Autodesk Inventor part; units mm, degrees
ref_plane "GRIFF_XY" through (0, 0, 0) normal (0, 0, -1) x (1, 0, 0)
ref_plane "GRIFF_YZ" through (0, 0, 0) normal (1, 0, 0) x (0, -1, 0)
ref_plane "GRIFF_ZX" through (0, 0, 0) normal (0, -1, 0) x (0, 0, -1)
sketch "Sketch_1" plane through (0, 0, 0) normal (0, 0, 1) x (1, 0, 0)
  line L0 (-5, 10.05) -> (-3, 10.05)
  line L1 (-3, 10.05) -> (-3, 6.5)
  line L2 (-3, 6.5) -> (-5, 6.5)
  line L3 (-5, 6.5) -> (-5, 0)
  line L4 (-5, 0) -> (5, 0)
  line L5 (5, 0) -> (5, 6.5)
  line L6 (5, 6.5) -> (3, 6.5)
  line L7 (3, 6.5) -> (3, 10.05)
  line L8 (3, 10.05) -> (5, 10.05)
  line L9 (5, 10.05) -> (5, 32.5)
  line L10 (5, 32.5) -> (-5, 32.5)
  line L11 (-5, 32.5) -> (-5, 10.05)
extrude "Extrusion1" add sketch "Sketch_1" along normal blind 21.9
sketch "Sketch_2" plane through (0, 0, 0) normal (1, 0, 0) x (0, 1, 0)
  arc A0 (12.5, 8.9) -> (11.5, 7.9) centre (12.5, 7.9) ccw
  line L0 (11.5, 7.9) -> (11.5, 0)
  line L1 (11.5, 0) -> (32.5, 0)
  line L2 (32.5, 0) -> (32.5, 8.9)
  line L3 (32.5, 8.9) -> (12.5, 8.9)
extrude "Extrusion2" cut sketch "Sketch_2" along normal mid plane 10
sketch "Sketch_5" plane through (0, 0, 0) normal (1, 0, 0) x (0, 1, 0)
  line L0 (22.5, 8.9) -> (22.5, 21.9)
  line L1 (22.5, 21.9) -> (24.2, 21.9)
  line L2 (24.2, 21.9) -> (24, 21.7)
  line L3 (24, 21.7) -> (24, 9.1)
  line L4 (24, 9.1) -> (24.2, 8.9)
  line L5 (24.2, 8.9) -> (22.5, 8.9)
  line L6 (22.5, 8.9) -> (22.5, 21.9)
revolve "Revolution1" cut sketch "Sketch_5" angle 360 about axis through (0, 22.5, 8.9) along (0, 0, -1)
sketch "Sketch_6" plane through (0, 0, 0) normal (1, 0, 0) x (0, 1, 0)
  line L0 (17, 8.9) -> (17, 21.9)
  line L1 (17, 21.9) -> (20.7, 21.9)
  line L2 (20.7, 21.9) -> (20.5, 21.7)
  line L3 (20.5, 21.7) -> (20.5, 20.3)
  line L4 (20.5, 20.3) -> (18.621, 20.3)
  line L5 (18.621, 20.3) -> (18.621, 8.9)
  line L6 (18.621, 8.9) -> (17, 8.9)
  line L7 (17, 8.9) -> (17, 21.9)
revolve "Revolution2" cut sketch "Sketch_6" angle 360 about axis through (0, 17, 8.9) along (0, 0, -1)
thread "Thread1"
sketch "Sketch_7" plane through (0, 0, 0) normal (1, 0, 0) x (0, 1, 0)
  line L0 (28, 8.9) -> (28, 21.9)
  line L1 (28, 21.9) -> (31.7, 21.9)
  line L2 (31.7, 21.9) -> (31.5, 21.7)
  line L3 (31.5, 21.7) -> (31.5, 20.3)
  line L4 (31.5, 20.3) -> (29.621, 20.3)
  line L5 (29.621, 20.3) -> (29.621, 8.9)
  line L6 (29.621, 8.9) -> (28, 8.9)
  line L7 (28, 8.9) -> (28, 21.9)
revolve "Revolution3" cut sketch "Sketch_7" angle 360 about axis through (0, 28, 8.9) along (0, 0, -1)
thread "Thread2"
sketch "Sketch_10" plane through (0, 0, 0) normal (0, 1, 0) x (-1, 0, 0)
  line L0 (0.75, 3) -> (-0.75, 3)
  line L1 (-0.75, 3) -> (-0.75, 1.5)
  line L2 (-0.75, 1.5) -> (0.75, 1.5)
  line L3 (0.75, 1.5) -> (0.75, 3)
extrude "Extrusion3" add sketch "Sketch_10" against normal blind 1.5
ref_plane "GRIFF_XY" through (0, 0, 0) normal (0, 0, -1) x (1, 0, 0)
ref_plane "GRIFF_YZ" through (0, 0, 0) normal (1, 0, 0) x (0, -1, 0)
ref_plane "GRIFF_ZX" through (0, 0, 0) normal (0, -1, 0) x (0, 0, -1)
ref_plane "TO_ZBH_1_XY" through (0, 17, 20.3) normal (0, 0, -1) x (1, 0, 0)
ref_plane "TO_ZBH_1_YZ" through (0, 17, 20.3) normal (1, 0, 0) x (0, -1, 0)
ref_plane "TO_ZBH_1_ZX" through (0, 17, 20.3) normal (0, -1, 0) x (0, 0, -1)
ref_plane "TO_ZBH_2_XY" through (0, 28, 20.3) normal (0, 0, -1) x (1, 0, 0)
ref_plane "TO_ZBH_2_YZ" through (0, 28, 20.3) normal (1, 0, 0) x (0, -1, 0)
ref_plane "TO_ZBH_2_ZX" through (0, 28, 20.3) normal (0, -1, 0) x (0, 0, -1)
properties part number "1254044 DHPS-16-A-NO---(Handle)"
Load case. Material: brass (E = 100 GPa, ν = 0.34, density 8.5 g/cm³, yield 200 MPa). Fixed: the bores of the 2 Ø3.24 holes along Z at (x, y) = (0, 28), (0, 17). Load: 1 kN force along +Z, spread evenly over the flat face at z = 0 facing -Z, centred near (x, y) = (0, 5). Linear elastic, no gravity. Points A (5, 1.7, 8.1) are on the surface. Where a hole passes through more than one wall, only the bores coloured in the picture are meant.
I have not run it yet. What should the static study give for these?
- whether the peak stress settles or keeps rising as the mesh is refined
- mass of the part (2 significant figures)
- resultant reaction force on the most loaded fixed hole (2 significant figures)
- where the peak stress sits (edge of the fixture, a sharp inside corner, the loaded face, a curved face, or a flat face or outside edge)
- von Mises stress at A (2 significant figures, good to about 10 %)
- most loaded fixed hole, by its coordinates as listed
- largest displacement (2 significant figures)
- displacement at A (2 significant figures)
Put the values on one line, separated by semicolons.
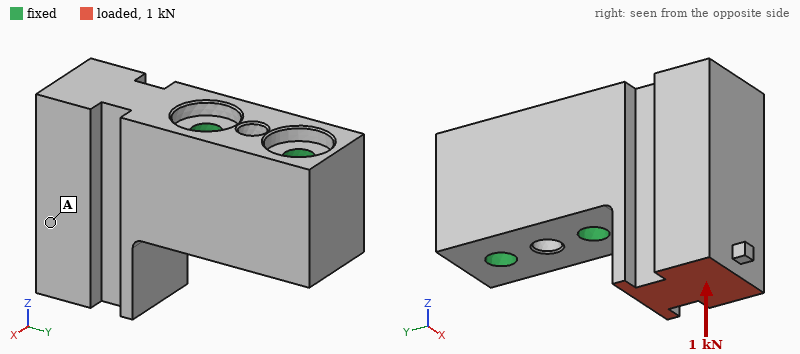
keeps rising; 39 g; 1.1 kN; edge of the fixture; 11 MPa; (0, 17); 16 µm; 11 µm
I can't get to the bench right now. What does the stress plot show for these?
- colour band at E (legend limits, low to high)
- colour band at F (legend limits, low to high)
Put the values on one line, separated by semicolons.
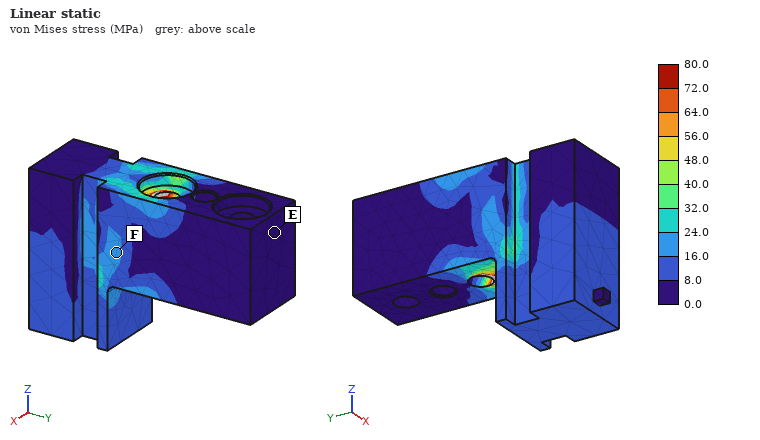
0.0 to 8.0 MPa; 16.0 to 24.0 MPa
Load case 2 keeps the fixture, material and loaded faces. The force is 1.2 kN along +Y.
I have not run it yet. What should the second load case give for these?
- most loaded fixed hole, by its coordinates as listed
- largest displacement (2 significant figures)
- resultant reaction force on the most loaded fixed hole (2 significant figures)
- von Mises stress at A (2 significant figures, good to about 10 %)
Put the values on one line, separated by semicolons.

(0, 17); 39 µm; 1.2 kN; 27 MPa
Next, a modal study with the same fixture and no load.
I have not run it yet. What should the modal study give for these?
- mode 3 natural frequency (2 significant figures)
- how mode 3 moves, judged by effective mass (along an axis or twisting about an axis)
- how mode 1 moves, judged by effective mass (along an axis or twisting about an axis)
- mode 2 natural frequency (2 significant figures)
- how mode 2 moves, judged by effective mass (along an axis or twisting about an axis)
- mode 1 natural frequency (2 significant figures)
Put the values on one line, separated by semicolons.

14 kHz; twisting about Y; along X; 11 kHz; along Z; 8300 Hz
